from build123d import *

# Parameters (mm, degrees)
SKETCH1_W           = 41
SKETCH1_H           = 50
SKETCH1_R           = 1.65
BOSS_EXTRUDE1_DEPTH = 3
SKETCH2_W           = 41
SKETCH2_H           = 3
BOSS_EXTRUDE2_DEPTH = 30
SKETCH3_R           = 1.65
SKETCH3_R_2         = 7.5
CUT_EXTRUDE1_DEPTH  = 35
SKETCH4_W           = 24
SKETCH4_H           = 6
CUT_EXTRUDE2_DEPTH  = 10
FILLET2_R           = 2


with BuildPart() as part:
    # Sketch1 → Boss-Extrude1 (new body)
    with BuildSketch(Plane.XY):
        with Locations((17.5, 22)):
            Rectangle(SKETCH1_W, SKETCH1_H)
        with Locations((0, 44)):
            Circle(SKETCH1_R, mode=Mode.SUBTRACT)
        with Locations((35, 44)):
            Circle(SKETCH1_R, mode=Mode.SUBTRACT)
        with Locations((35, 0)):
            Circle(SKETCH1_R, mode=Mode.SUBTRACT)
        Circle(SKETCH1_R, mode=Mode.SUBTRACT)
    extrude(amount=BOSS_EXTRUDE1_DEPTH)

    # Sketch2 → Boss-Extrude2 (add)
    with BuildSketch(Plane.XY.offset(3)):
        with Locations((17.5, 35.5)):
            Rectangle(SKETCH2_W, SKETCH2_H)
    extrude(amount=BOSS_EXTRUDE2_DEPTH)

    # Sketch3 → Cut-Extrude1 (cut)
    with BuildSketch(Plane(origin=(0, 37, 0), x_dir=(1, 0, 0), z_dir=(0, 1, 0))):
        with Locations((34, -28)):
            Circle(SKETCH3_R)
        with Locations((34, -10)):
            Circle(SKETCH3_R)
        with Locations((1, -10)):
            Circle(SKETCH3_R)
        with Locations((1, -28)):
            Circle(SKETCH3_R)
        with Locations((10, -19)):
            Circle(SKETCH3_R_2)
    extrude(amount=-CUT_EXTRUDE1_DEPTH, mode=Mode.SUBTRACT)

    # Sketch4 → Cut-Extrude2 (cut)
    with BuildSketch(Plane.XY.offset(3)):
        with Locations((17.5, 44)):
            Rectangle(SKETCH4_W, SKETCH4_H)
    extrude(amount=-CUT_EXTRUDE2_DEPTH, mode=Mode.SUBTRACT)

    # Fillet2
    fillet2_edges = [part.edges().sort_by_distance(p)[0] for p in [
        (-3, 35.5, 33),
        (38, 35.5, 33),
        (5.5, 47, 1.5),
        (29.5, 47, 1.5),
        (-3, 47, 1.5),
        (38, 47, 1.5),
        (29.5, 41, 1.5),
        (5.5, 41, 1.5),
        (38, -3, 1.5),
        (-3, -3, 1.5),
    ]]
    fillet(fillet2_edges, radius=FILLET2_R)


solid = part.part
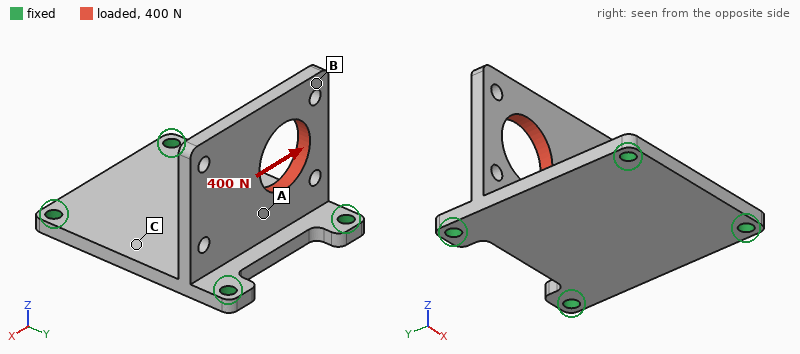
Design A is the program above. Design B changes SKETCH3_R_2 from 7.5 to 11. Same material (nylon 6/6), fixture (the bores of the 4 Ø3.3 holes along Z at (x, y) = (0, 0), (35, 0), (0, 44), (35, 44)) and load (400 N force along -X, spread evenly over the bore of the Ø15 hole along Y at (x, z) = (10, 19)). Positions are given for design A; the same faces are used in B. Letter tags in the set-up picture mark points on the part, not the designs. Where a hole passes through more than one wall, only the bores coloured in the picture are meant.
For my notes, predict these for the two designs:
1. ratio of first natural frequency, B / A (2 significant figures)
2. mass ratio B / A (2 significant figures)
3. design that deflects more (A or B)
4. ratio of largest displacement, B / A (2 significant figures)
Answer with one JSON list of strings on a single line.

["0.98", "0.93", "B", "1.5"]
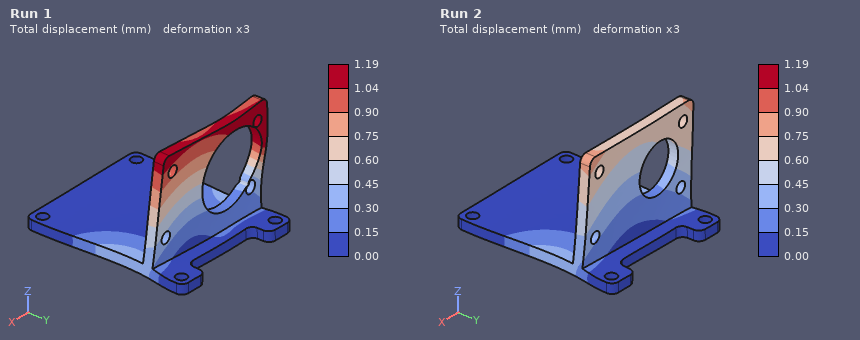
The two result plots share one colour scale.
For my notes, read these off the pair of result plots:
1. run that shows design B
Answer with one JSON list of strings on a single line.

["Run 1"]
